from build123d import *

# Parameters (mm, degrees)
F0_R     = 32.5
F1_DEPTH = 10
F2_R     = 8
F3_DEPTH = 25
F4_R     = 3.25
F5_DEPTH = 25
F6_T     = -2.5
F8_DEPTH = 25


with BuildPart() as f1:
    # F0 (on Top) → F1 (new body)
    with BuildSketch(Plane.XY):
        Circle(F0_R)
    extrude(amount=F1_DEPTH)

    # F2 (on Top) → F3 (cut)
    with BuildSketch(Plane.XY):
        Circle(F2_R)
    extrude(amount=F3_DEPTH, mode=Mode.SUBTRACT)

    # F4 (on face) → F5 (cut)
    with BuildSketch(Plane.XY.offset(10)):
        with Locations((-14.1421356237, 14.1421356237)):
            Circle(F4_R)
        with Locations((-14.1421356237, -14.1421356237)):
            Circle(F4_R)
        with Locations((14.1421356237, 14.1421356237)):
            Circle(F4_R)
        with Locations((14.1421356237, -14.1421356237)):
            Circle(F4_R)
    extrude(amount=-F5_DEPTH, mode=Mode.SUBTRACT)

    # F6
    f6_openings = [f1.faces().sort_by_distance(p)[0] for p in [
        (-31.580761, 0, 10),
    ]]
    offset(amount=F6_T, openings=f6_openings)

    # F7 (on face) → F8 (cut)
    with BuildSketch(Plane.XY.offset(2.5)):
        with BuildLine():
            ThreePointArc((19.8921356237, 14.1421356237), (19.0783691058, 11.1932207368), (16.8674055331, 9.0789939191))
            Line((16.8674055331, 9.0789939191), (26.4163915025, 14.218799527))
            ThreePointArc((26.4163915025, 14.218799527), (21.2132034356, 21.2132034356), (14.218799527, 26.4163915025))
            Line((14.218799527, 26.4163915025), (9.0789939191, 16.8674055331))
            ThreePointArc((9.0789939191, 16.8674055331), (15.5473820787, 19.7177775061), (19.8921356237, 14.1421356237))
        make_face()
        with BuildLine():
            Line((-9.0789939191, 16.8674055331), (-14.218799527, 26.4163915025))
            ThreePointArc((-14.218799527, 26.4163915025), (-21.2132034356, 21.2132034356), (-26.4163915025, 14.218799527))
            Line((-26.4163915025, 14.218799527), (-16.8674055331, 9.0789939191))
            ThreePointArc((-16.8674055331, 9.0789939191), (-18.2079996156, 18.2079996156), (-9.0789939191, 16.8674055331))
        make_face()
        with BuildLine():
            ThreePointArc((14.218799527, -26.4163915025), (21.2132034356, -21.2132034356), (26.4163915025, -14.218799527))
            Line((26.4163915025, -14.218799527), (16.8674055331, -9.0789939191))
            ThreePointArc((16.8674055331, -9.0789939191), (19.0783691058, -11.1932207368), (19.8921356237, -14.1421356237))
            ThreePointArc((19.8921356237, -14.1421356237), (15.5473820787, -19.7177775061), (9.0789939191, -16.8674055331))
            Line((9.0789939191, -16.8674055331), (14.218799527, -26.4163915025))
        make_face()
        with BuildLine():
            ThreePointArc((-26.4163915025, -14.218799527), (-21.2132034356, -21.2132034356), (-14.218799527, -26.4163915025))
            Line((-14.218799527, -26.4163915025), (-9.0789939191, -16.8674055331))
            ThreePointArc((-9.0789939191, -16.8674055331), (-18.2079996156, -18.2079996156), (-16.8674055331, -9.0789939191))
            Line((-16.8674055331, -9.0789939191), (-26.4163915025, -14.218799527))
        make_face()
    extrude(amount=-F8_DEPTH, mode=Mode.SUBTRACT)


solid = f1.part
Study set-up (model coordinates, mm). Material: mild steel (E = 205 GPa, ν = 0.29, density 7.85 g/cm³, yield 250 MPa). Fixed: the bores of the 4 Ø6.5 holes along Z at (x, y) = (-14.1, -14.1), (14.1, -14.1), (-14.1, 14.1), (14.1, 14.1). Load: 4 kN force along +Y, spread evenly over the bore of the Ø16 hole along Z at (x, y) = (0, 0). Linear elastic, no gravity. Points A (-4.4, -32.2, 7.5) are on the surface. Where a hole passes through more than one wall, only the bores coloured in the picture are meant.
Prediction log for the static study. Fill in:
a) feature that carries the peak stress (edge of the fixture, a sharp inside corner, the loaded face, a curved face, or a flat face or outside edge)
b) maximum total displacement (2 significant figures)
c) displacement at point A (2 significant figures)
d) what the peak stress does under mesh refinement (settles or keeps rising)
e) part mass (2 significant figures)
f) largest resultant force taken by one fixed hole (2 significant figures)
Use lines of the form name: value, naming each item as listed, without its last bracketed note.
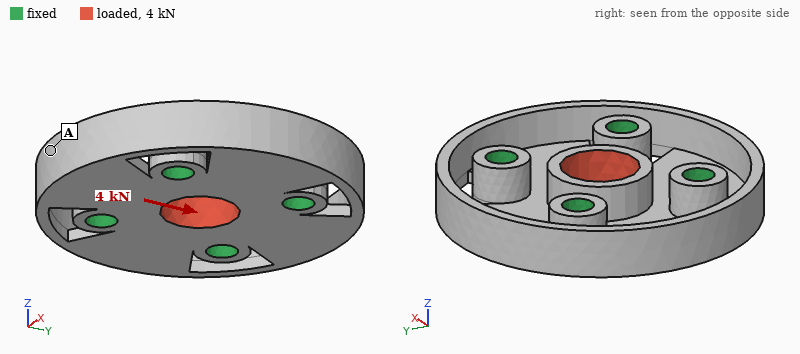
feature that carries the peak stress: edge of the fixture
maximum total displacement: 9.9 µm
displacement at point A: 2.0 µm
what the peak stress does under mesh refinement: keeps rising
part mass: 110 g
largest resultant force taken by one fixed hole: 1.1 kN
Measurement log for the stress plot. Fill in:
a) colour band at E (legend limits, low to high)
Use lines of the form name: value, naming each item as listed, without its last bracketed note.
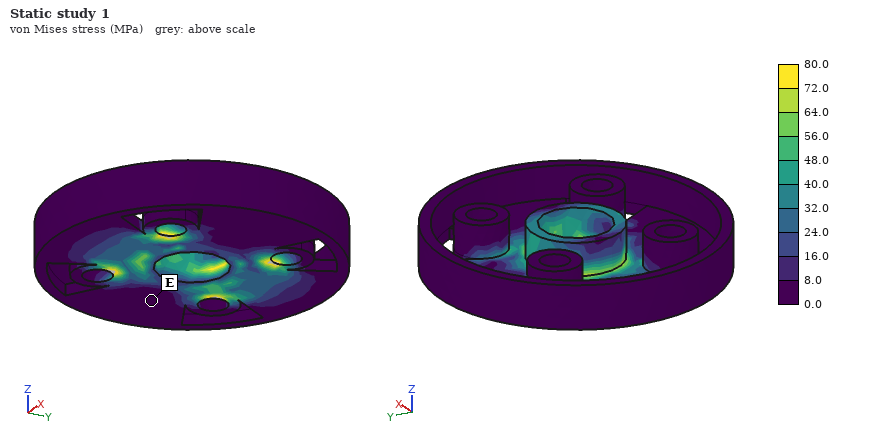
colour band at E: 0.0 to 8.0 MPa
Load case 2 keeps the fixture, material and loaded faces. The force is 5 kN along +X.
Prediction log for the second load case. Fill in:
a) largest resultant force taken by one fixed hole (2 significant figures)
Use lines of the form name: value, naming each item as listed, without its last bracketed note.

largest resultant force taken by one fixed hole: 1.3 kN
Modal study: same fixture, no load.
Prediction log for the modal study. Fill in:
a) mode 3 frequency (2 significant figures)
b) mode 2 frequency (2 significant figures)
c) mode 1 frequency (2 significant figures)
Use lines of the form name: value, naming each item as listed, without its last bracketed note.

mode 3 frequency: 4500 Hz
mode 2 frequency: 3900 Hz
mode 1 frequency: 3900 Hz
